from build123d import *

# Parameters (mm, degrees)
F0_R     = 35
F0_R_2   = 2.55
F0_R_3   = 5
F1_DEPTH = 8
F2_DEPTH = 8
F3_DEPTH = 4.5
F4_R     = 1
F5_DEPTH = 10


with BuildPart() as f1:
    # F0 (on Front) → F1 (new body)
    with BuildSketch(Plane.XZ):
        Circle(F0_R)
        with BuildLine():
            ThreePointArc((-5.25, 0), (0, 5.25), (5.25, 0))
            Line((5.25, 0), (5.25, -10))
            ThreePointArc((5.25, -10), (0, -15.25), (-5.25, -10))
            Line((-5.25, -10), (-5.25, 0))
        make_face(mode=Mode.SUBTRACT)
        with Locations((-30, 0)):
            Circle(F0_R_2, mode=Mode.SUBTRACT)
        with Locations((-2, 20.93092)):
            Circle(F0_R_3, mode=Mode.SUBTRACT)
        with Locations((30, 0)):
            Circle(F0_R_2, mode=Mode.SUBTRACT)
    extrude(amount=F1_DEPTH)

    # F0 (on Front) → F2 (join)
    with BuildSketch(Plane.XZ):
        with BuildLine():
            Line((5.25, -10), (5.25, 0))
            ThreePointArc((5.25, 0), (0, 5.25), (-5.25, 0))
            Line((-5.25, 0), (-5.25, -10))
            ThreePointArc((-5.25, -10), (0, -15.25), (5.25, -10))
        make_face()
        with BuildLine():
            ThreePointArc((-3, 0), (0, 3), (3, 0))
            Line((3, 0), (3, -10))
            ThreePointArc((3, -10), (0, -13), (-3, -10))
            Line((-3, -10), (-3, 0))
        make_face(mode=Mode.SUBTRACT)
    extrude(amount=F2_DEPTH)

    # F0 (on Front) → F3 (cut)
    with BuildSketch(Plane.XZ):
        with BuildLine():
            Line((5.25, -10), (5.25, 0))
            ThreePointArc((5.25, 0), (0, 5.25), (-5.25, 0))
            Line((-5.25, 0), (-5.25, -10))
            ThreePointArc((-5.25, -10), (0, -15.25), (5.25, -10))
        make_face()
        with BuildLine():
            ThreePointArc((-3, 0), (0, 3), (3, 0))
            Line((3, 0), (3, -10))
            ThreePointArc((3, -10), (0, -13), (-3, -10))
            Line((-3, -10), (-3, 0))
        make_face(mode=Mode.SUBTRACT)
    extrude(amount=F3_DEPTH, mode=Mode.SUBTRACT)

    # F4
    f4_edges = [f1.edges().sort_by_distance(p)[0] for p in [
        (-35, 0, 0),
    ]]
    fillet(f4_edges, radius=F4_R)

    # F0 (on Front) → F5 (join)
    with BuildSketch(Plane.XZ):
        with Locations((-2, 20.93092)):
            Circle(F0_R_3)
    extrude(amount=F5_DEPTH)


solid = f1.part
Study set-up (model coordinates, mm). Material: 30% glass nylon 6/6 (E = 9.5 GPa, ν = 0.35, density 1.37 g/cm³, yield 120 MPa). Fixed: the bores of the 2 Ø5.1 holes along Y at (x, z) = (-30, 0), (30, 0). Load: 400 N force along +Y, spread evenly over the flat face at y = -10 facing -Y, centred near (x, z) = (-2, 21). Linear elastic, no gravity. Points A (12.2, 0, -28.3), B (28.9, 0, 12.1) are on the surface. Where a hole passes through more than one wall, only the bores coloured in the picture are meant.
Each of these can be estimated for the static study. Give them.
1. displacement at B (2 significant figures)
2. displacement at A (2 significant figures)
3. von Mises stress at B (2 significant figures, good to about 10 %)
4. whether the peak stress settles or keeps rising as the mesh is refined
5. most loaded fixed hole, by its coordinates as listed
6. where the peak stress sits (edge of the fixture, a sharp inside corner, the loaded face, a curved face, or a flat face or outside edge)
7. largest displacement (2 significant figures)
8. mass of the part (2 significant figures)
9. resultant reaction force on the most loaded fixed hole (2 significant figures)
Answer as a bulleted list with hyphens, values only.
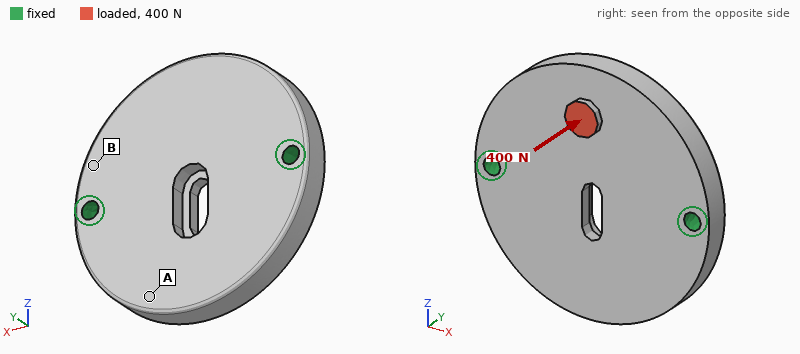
- 0.036 mm
- 0.054 mm
- 10.0 MPa
- keeps rising
- (-30, 0)
- edge of the fixture
- 0.24 mm
- 40 g
- 220 N
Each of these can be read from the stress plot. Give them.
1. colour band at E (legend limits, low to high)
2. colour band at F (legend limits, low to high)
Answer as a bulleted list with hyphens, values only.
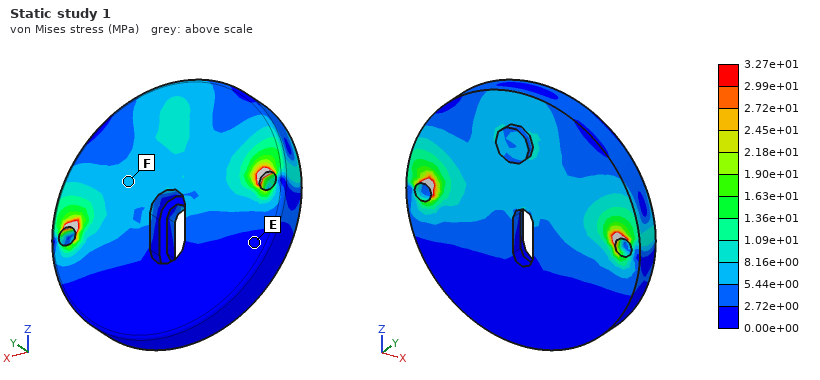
- 0.00e+00 to 2.72e+00 MPa
- 5.44e+00 to 8.16e+00 MPa
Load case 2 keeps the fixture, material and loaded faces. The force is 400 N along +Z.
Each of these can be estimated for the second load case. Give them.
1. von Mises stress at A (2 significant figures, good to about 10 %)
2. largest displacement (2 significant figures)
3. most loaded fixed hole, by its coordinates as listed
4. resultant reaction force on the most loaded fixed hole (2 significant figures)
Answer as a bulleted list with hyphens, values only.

- 0.96 MPa
- 82 µm
- (-30, 0)
- 220 N
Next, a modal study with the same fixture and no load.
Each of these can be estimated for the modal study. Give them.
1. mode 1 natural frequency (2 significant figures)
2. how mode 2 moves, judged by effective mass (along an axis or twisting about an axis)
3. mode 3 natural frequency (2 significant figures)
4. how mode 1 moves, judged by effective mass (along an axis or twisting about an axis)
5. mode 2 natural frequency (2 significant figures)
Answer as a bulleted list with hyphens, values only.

- 2100 Hz
- along Y
- 6100 Hz
- twisting about X
- 2800 Hz
